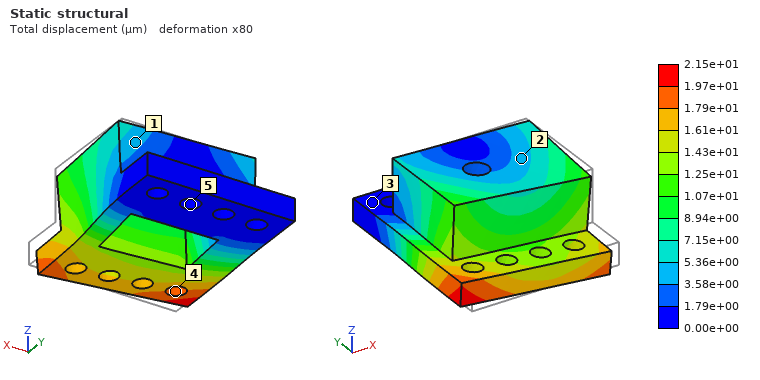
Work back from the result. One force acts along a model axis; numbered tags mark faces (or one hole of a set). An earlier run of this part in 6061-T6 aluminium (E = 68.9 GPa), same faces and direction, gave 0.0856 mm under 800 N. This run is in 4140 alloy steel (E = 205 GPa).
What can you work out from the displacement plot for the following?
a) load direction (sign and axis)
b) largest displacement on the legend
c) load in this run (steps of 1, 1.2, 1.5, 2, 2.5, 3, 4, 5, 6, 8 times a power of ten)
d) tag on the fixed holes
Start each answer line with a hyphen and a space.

- -X
- 2.15e+01 µm
- 600 N
- 5
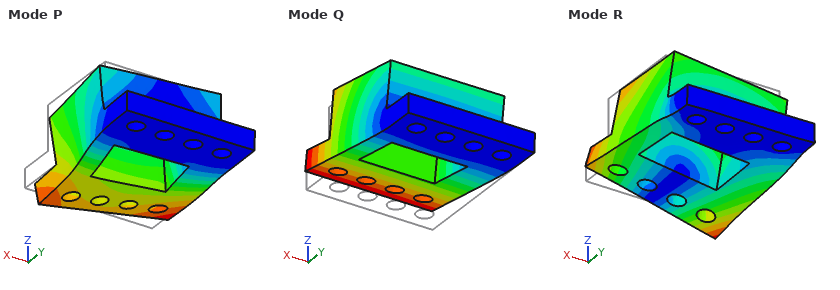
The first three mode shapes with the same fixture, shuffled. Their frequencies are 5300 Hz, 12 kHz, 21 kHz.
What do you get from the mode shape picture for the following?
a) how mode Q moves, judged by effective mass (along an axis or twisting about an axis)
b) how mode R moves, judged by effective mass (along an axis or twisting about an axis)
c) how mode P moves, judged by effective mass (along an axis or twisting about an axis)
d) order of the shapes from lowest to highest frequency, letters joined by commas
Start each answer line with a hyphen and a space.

- along Z
- along X
- along X
- Q, P, R
